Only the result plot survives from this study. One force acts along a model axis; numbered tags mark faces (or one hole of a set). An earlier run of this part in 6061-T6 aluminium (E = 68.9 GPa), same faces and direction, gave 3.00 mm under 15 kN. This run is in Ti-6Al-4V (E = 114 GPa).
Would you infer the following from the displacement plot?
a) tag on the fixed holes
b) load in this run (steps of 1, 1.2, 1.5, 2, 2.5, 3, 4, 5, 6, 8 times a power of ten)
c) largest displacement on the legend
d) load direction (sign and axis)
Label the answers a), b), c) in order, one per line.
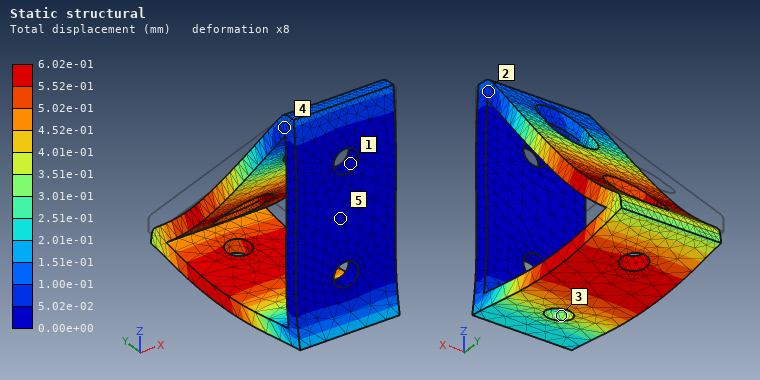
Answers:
a) 1
b) 5 kN
c) 6.02e-01 mm
d) -Z
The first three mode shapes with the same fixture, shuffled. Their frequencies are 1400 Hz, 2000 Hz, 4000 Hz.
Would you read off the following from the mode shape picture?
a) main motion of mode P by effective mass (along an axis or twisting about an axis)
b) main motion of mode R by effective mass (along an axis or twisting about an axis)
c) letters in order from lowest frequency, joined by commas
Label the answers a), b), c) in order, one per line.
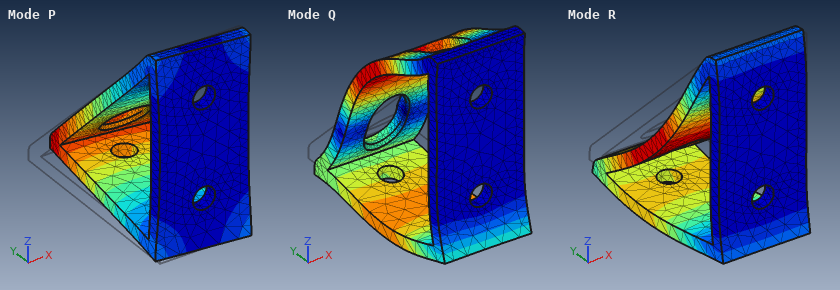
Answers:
a) along X
b) along Z
c) P, R, Q
